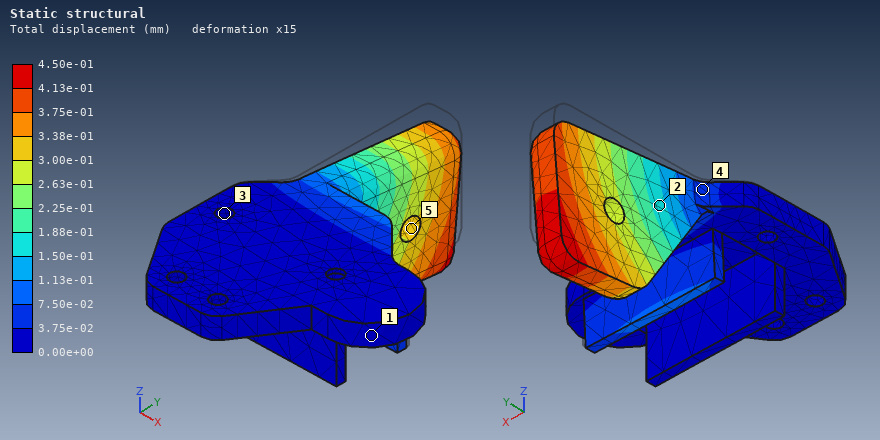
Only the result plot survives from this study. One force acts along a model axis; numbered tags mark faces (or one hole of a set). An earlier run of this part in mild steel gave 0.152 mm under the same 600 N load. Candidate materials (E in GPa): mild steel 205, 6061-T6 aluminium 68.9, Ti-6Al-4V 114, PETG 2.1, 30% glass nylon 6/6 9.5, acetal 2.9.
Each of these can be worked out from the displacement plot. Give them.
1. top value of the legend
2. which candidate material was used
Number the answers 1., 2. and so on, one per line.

1. 4.50e-01 mm
2. 6061-T6 aluminium
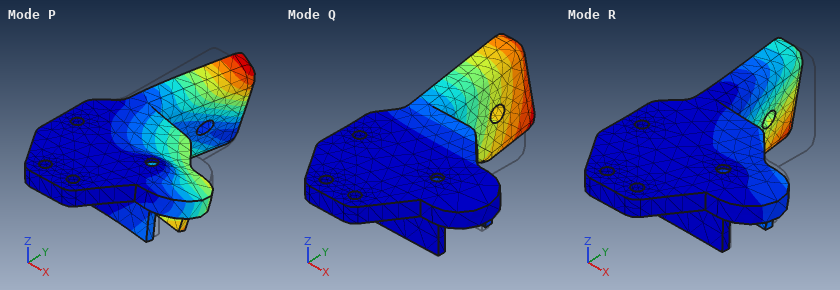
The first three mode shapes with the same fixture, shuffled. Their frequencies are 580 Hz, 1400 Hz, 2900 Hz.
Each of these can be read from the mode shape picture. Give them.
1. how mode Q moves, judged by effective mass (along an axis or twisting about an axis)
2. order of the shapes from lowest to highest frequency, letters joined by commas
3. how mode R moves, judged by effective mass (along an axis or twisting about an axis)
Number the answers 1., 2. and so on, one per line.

1. along Z
2. Q, R, P
3. along X
